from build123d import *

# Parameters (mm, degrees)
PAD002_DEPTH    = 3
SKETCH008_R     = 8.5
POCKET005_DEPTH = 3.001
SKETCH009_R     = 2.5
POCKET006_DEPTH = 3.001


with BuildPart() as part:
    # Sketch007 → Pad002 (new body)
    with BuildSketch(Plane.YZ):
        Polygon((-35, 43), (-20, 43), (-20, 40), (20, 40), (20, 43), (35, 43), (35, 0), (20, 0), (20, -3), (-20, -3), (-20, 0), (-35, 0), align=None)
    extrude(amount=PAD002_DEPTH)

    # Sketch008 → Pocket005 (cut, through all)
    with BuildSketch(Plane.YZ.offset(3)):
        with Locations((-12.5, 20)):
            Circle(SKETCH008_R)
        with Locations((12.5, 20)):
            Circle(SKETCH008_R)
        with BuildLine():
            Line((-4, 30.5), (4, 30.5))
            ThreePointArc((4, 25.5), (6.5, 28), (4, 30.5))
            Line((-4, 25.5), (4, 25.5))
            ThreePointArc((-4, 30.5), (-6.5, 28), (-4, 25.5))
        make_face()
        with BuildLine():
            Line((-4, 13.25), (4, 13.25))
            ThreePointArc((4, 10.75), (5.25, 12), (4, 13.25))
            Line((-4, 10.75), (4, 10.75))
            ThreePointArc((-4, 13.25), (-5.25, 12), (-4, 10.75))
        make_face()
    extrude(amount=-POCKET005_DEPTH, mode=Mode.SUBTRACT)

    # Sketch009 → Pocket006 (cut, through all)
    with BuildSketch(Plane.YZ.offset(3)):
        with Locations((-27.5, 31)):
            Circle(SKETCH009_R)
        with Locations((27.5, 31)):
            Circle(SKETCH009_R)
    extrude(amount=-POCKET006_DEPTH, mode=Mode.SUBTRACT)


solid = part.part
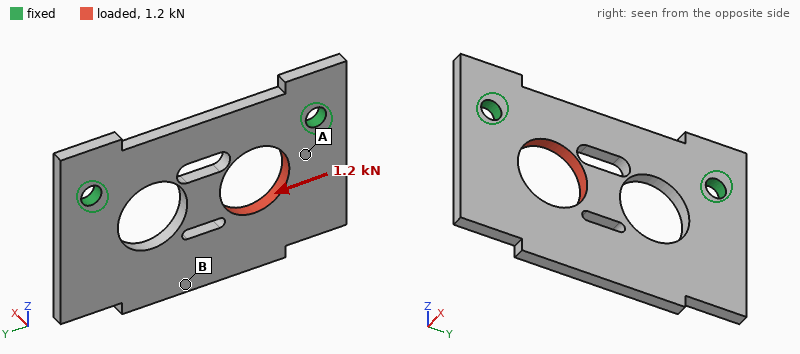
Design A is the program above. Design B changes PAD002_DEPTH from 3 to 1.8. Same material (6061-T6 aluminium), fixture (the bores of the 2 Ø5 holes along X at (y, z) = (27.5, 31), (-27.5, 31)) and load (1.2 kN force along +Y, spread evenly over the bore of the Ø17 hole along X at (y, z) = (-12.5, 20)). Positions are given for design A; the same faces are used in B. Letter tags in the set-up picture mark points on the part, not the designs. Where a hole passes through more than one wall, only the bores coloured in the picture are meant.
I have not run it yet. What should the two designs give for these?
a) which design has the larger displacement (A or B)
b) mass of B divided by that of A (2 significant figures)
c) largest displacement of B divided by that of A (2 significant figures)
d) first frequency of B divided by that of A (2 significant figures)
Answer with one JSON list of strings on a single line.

["B", "0.60", "1.7", "0.62"]
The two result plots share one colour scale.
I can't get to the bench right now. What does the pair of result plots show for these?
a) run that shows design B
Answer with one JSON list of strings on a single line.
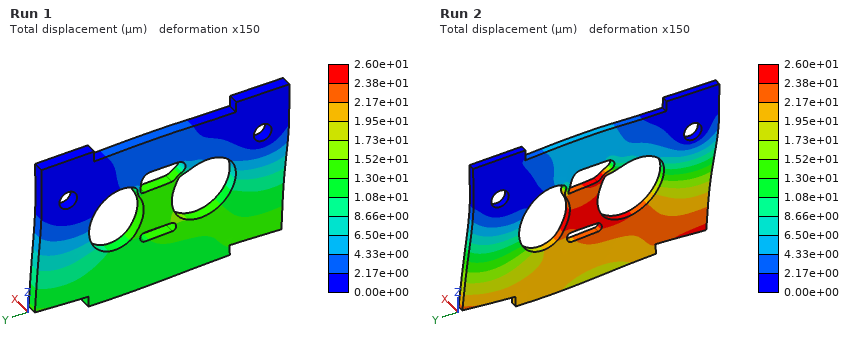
["Run 2"]
